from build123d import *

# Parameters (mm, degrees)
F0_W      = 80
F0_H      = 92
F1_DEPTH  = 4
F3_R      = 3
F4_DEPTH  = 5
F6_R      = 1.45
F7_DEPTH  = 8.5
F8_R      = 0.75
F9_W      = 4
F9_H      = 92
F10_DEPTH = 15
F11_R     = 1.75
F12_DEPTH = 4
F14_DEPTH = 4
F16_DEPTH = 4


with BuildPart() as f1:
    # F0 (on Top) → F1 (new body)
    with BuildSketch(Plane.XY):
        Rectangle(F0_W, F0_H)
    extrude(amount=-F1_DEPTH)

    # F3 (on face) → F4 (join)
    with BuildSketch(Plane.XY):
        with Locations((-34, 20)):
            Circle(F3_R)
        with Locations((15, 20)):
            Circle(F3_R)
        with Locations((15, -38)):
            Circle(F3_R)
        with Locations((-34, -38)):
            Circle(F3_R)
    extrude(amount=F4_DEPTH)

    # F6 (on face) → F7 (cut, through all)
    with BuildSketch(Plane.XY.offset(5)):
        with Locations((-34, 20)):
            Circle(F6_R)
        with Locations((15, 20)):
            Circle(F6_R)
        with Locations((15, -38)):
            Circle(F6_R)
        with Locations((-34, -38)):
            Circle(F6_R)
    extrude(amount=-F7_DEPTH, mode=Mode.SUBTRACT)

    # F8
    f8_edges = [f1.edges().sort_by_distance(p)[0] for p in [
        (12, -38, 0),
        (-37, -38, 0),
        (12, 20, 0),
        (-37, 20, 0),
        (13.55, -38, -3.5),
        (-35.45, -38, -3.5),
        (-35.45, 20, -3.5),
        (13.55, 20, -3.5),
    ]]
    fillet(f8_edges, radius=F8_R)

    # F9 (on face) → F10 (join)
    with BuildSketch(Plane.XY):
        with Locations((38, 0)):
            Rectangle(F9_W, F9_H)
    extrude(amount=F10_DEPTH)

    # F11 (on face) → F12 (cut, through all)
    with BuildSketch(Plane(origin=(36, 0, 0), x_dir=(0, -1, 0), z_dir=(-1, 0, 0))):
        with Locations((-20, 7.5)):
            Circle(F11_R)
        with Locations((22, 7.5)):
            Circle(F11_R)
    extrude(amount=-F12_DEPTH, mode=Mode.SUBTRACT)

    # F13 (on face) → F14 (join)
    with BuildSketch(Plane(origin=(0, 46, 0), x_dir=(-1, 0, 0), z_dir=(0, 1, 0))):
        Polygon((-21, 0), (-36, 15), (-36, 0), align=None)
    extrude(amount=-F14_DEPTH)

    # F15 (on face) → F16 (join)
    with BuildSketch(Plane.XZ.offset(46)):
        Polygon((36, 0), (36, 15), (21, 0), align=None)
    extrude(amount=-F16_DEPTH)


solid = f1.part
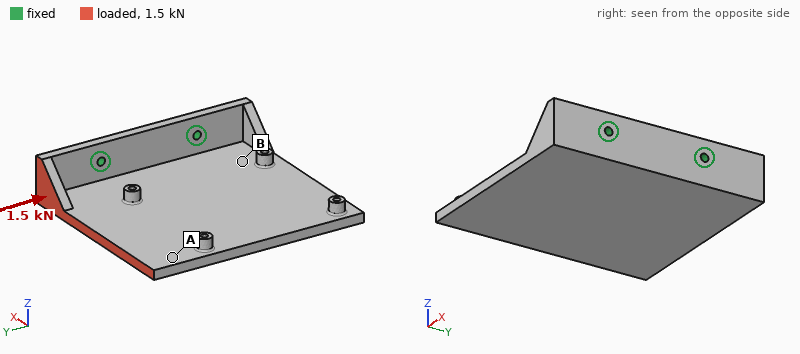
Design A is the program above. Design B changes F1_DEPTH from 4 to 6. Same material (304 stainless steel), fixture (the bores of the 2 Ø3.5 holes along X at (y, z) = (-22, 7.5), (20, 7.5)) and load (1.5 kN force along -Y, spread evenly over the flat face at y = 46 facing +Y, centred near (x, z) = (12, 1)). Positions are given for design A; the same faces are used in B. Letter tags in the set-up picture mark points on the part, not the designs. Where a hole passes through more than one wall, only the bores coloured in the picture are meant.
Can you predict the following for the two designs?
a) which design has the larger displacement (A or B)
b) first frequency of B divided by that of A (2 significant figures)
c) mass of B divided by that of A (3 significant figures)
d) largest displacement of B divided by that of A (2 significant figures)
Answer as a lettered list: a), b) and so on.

a) A
b) 1.0
c) 1.41
d) 0.83
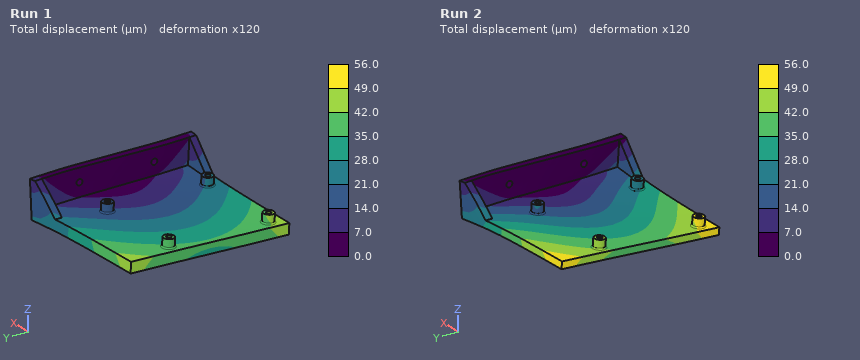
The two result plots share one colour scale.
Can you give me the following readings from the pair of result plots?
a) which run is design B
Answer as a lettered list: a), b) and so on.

a) Run 1
